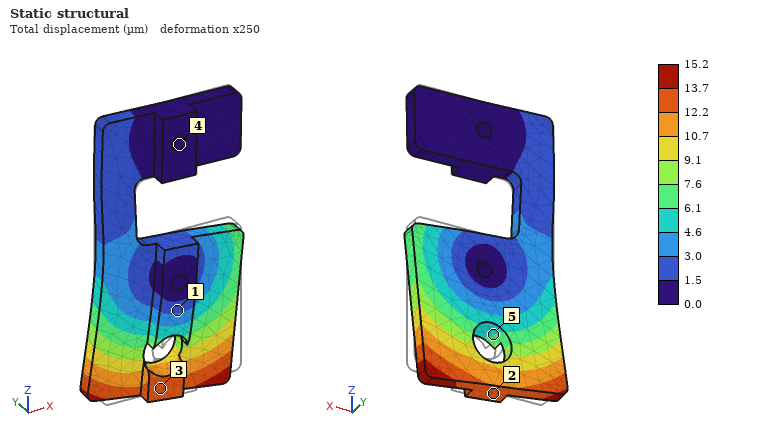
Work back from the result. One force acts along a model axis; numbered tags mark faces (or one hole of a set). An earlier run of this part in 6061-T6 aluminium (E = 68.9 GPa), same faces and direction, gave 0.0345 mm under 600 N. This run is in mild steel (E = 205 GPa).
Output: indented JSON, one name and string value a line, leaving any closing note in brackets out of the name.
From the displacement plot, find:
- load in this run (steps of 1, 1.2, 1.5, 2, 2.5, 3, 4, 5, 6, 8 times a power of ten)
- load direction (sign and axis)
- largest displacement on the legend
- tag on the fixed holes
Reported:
{
  "load in this run": "800 N",
  "load direction": "-X",
  "largest displacement on the legend": "15.2 µm",
  "tag on the fixed holes": "4"
}
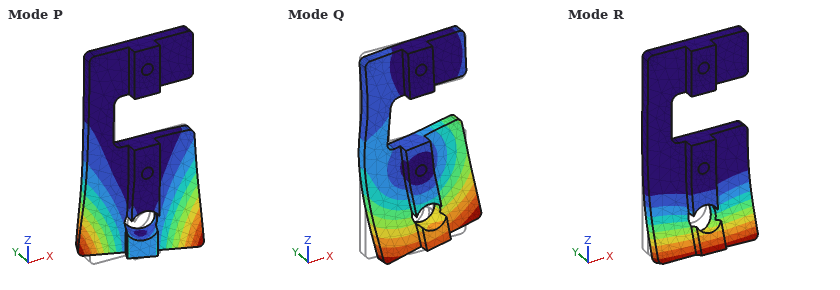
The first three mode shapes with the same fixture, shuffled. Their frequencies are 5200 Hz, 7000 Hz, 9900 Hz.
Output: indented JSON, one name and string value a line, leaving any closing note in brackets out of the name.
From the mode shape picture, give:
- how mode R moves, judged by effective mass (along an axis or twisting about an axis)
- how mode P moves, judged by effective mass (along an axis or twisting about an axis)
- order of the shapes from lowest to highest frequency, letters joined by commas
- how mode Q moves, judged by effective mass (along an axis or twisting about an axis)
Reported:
{
  "how mode R moves, judged by effective mass": "along Y",
  "how mode P moves, judged by effective mass": "twisting about Z",
  "order of the shapes from lowest to highest frequency, letters joined by commas": "R, P, Q",
  "how mode Q moves, judged by effective mass": "along X"
}
